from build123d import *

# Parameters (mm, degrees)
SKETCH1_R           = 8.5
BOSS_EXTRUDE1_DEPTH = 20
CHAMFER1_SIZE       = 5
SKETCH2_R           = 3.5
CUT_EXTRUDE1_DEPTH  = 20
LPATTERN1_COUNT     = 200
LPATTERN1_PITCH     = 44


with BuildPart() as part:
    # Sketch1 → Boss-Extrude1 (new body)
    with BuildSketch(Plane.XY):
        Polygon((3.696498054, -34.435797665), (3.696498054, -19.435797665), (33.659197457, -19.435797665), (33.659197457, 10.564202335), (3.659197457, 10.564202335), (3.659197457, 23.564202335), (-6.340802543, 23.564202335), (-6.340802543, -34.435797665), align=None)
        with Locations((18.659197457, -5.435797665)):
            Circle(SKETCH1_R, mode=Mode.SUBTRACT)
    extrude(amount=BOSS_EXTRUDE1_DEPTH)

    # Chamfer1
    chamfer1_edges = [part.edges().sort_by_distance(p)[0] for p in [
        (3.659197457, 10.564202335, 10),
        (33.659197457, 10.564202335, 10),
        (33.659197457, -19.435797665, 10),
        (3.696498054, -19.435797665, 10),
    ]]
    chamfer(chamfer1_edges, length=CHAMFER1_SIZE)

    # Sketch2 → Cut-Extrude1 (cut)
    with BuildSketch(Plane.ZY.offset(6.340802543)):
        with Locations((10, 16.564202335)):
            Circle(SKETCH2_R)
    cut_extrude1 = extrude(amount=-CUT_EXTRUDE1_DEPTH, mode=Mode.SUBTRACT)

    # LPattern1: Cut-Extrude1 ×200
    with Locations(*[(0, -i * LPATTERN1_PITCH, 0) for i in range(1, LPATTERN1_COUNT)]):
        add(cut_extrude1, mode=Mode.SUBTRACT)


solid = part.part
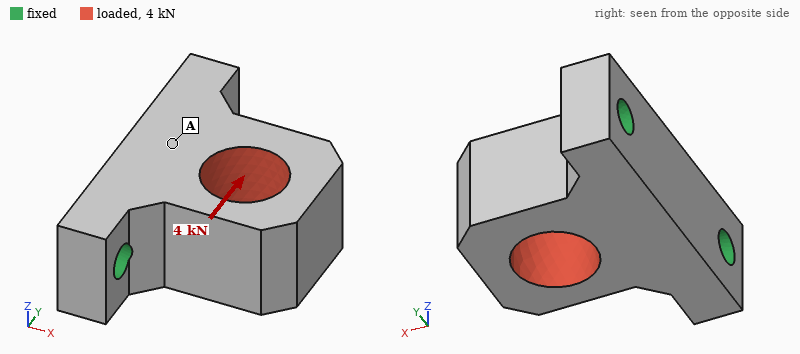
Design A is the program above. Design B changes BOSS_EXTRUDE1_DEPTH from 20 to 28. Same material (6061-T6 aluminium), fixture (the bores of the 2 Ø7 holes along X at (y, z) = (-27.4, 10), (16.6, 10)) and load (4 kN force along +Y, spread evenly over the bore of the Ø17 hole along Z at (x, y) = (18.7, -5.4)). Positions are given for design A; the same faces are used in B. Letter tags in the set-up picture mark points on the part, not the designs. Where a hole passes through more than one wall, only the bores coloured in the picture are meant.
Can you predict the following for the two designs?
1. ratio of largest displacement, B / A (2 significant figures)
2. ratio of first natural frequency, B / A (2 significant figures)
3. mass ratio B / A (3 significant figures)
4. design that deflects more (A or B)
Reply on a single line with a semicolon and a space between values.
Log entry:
0.78; 0.93; 1.41; A
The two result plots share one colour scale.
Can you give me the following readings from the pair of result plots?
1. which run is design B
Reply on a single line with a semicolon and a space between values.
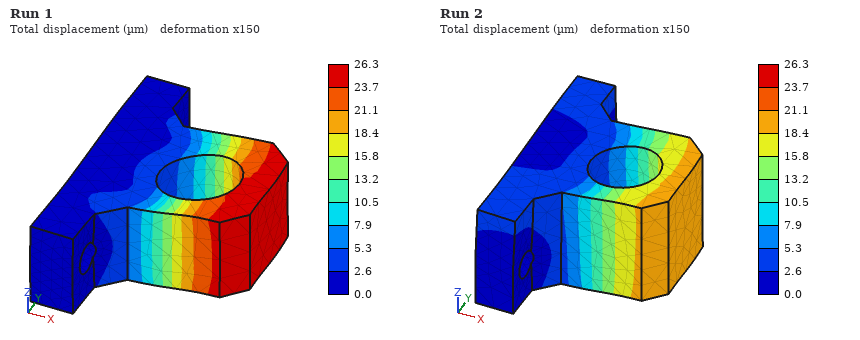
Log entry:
Run 2
